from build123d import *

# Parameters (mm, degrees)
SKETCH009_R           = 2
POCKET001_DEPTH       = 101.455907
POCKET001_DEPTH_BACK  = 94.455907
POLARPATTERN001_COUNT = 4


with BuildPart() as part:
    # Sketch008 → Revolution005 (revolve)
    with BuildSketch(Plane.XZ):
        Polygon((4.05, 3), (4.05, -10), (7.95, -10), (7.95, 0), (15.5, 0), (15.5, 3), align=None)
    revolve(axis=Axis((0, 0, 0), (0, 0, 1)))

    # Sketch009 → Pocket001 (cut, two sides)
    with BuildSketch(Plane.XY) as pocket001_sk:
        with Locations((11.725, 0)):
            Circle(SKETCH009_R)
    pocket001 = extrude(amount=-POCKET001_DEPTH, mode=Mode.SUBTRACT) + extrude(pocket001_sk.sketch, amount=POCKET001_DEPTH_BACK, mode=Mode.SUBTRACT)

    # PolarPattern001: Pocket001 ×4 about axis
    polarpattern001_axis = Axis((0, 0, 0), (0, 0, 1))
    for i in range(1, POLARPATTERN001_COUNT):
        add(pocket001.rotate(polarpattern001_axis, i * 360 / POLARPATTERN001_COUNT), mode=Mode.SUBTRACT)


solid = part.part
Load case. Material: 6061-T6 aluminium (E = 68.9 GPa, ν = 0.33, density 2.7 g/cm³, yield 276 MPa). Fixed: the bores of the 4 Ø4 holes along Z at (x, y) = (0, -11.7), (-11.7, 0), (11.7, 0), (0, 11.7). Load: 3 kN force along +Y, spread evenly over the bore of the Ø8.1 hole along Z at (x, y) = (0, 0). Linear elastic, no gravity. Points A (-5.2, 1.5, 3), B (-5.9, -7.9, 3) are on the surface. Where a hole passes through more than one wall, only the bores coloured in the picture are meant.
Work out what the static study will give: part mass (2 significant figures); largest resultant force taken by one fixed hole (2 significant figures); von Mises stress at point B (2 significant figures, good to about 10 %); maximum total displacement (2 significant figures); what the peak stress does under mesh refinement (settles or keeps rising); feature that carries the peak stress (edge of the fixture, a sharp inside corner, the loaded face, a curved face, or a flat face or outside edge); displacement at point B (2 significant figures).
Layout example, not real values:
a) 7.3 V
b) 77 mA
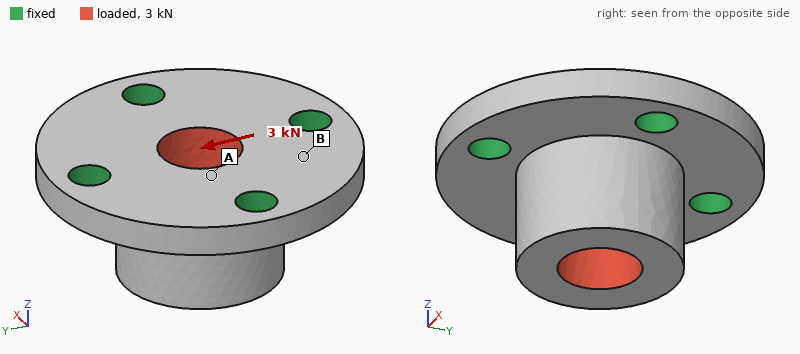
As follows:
a) 9.3 g
b) 1.2 kN
c) 19 MPa
d) 18 µm
e) keeps rising
f) edge of the fixture
g) 4.2 µm
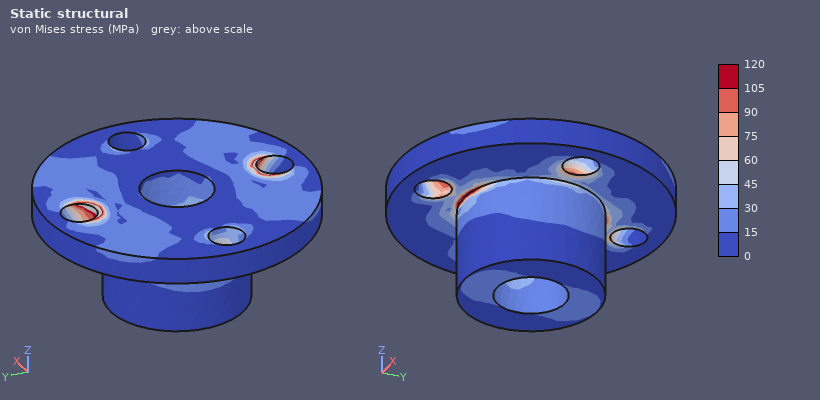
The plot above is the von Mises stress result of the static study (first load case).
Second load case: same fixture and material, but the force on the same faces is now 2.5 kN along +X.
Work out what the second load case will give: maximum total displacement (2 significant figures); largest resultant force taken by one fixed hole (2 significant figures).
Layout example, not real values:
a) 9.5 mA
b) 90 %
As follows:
a) 15 µm
b) 1.0 kN
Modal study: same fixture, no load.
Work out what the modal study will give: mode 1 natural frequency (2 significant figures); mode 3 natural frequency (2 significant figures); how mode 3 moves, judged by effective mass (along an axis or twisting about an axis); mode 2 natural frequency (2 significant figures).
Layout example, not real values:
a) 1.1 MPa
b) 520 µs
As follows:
a) 32 kHz
b) 40 kHz
c) along Z
d) 32 kHz
